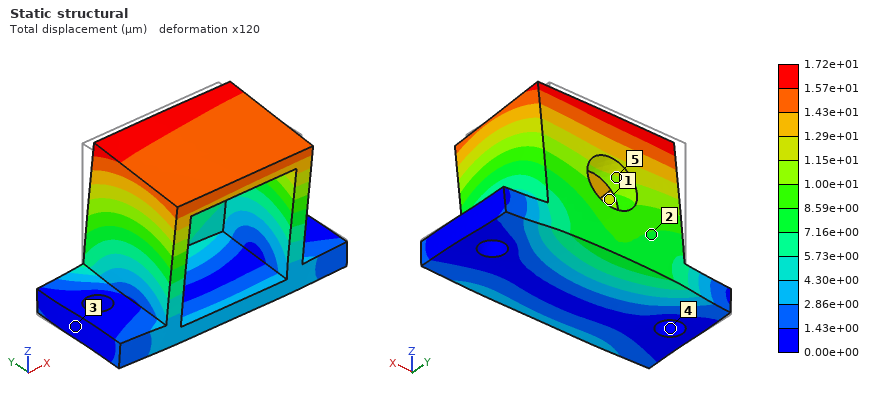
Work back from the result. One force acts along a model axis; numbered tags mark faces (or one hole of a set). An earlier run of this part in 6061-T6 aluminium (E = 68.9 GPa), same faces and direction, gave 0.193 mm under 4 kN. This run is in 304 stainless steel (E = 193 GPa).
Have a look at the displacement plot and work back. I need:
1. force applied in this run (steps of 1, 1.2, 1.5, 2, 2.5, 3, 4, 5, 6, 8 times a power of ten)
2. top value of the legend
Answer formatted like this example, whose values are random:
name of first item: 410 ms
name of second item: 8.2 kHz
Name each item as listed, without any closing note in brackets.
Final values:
force applied in this run: 1 kN
top value of the legend: 1.72e+01 µm
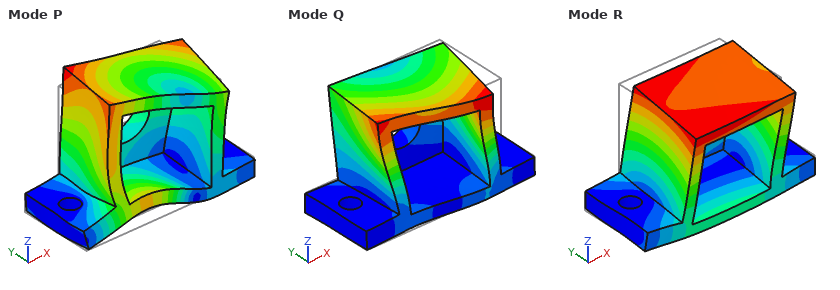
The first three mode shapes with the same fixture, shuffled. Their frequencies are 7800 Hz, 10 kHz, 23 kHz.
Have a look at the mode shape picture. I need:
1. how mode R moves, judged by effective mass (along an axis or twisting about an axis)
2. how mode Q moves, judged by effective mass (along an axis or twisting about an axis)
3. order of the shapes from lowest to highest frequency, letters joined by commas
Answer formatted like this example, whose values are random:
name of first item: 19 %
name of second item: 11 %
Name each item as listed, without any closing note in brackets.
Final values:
how mode R moves, judged by effective mass: along Y
how mode Q moves, judged by effective mass: along X
order of the shapes from lowest to highest frequency, letters joined by commas: R, Q, P
